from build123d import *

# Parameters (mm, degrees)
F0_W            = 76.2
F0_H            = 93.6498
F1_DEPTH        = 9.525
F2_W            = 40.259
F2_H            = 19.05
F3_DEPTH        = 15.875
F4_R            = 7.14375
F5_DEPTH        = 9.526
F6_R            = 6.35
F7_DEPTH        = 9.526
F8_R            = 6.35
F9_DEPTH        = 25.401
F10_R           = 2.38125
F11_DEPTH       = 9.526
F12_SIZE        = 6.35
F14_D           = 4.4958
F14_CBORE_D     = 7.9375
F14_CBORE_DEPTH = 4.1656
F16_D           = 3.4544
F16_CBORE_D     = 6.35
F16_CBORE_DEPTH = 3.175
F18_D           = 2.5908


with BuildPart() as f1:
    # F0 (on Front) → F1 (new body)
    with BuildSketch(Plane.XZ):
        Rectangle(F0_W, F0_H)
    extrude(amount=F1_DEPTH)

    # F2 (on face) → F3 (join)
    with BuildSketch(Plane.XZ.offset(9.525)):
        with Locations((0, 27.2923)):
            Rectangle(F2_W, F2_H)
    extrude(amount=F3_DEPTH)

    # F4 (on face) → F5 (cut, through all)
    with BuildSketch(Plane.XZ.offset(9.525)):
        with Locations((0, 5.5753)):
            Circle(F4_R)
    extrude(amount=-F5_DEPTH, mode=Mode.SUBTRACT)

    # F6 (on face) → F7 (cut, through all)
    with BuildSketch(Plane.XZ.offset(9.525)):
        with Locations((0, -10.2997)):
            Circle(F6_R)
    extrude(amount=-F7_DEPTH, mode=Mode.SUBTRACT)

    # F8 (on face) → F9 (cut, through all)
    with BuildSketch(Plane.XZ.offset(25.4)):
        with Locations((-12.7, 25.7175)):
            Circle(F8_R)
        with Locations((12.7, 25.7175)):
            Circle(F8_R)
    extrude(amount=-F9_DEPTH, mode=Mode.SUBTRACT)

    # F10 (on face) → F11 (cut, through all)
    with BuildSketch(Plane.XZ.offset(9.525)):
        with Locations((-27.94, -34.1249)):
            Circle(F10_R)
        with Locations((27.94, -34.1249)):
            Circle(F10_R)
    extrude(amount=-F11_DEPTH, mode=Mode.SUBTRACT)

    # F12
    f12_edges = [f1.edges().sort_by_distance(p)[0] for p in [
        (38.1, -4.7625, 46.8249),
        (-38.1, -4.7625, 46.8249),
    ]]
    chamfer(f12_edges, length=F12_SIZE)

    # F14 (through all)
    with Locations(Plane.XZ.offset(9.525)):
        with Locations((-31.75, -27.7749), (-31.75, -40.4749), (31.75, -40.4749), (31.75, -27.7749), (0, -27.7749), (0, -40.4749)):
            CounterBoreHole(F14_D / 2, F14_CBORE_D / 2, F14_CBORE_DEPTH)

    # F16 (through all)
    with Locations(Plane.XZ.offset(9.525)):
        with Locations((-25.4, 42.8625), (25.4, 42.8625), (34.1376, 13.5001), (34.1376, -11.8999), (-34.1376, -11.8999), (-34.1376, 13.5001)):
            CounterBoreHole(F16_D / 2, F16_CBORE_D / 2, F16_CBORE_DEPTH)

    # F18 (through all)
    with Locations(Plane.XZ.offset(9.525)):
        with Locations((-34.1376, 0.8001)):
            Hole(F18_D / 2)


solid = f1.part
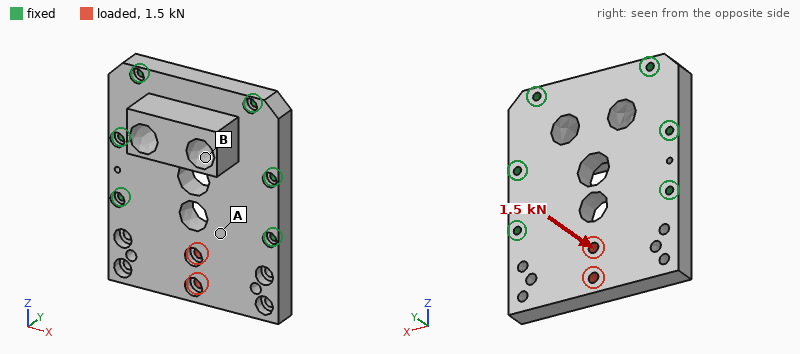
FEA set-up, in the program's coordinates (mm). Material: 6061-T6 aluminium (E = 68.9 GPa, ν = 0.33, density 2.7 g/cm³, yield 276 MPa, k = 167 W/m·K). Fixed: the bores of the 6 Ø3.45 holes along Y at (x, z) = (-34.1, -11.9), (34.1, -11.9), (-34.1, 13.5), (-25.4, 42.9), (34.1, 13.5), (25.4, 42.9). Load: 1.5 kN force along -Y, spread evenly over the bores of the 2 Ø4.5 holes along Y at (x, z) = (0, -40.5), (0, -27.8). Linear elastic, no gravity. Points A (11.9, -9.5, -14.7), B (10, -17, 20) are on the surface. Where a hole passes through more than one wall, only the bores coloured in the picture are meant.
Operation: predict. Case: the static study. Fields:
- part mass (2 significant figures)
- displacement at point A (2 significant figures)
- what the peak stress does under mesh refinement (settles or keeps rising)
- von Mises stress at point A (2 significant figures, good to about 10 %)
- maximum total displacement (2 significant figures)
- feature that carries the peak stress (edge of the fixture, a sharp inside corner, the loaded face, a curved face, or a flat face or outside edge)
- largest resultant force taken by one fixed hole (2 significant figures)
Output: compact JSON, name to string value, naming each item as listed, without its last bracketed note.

{"part mass": "180 g", "displacement at point A": "0.031 mm", "what the peak stress does under mesh refinement": "keeps rising", "von Mises stress at point A": "27 MPa", "maximum total displacement": "0.12 mm", "feature that carries the peak stress": "edge of the fixture", "largest resultant force taken by one fixed hole": "1.3 kN"}
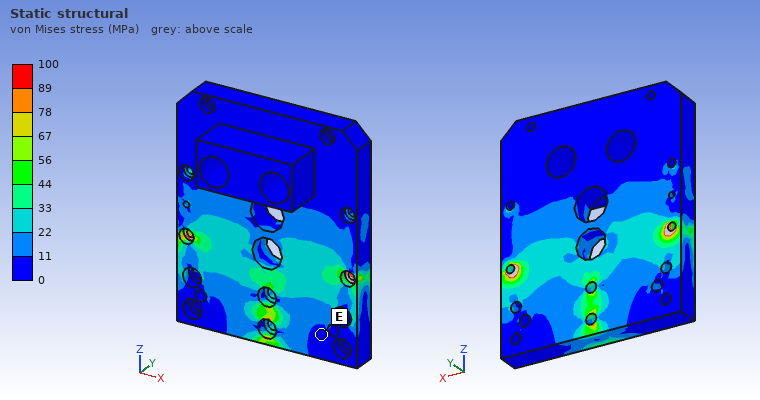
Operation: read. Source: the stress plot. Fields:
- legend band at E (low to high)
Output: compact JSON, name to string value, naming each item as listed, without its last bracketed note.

{"legend band at E": "0 to 11 MPa"}
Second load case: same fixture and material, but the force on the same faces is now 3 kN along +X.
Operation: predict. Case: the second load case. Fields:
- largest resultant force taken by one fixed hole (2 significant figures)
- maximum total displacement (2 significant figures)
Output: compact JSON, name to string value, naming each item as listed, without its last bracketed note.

{"largest resultant force taken by one fixed hole": "1.5 kN", "maximum total displacement": "12 µm"}
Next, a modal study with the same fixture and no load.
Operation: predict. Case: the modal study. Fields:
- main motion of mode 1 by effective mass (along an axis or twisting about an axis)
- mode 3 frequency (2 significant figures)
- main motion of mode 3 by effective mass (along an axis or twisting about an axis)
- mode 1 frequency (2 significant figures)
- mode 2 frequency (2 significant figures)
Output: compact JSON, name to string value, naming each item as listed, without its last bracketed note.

{"main motion of mode 1 by effective mass": "along Y", "mode 3 frequency": "8200 Hz", "main motion of mode 3 by effective mass": "along Y", "mode 1 frequency": "3600 Hz", "mode 2 frequency": "7200 Hz"}
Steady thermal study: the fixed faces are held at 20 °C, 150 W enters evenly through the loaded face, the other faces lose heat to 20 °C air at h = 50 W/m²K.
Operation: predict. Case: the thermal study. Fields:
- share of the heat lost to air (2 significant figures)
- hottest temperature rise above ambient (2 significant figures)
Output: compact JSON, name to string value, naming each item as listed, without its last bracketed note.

{"share of the heat lost to air": "12 %", "hottest temperature rise above ambient": "78 K"}
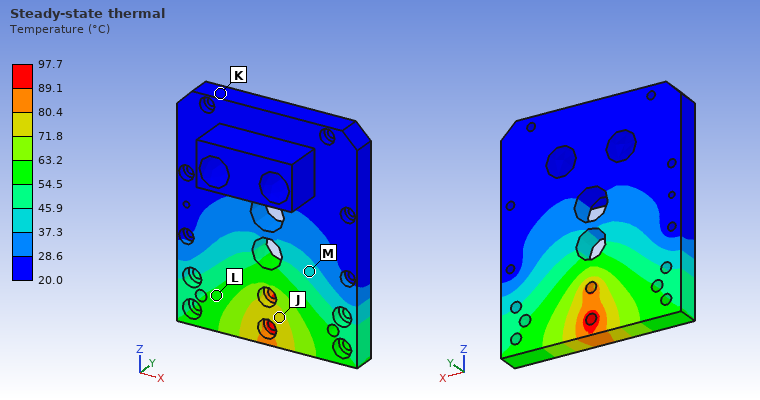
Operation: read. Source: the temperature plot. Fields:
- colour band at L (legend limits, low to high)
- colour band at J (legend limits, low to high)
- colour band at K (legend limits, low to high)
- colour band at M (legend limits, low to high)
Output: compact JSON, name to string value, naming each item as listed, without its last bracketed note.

{"colour band at L": "54.5 to 63.2 °C", "colour band at J": "71.8 to 80.4 °C", "colour band at K": "20.0 to 28.6 °C", "colour band at M": "37.3 to 45.9 °C"}
